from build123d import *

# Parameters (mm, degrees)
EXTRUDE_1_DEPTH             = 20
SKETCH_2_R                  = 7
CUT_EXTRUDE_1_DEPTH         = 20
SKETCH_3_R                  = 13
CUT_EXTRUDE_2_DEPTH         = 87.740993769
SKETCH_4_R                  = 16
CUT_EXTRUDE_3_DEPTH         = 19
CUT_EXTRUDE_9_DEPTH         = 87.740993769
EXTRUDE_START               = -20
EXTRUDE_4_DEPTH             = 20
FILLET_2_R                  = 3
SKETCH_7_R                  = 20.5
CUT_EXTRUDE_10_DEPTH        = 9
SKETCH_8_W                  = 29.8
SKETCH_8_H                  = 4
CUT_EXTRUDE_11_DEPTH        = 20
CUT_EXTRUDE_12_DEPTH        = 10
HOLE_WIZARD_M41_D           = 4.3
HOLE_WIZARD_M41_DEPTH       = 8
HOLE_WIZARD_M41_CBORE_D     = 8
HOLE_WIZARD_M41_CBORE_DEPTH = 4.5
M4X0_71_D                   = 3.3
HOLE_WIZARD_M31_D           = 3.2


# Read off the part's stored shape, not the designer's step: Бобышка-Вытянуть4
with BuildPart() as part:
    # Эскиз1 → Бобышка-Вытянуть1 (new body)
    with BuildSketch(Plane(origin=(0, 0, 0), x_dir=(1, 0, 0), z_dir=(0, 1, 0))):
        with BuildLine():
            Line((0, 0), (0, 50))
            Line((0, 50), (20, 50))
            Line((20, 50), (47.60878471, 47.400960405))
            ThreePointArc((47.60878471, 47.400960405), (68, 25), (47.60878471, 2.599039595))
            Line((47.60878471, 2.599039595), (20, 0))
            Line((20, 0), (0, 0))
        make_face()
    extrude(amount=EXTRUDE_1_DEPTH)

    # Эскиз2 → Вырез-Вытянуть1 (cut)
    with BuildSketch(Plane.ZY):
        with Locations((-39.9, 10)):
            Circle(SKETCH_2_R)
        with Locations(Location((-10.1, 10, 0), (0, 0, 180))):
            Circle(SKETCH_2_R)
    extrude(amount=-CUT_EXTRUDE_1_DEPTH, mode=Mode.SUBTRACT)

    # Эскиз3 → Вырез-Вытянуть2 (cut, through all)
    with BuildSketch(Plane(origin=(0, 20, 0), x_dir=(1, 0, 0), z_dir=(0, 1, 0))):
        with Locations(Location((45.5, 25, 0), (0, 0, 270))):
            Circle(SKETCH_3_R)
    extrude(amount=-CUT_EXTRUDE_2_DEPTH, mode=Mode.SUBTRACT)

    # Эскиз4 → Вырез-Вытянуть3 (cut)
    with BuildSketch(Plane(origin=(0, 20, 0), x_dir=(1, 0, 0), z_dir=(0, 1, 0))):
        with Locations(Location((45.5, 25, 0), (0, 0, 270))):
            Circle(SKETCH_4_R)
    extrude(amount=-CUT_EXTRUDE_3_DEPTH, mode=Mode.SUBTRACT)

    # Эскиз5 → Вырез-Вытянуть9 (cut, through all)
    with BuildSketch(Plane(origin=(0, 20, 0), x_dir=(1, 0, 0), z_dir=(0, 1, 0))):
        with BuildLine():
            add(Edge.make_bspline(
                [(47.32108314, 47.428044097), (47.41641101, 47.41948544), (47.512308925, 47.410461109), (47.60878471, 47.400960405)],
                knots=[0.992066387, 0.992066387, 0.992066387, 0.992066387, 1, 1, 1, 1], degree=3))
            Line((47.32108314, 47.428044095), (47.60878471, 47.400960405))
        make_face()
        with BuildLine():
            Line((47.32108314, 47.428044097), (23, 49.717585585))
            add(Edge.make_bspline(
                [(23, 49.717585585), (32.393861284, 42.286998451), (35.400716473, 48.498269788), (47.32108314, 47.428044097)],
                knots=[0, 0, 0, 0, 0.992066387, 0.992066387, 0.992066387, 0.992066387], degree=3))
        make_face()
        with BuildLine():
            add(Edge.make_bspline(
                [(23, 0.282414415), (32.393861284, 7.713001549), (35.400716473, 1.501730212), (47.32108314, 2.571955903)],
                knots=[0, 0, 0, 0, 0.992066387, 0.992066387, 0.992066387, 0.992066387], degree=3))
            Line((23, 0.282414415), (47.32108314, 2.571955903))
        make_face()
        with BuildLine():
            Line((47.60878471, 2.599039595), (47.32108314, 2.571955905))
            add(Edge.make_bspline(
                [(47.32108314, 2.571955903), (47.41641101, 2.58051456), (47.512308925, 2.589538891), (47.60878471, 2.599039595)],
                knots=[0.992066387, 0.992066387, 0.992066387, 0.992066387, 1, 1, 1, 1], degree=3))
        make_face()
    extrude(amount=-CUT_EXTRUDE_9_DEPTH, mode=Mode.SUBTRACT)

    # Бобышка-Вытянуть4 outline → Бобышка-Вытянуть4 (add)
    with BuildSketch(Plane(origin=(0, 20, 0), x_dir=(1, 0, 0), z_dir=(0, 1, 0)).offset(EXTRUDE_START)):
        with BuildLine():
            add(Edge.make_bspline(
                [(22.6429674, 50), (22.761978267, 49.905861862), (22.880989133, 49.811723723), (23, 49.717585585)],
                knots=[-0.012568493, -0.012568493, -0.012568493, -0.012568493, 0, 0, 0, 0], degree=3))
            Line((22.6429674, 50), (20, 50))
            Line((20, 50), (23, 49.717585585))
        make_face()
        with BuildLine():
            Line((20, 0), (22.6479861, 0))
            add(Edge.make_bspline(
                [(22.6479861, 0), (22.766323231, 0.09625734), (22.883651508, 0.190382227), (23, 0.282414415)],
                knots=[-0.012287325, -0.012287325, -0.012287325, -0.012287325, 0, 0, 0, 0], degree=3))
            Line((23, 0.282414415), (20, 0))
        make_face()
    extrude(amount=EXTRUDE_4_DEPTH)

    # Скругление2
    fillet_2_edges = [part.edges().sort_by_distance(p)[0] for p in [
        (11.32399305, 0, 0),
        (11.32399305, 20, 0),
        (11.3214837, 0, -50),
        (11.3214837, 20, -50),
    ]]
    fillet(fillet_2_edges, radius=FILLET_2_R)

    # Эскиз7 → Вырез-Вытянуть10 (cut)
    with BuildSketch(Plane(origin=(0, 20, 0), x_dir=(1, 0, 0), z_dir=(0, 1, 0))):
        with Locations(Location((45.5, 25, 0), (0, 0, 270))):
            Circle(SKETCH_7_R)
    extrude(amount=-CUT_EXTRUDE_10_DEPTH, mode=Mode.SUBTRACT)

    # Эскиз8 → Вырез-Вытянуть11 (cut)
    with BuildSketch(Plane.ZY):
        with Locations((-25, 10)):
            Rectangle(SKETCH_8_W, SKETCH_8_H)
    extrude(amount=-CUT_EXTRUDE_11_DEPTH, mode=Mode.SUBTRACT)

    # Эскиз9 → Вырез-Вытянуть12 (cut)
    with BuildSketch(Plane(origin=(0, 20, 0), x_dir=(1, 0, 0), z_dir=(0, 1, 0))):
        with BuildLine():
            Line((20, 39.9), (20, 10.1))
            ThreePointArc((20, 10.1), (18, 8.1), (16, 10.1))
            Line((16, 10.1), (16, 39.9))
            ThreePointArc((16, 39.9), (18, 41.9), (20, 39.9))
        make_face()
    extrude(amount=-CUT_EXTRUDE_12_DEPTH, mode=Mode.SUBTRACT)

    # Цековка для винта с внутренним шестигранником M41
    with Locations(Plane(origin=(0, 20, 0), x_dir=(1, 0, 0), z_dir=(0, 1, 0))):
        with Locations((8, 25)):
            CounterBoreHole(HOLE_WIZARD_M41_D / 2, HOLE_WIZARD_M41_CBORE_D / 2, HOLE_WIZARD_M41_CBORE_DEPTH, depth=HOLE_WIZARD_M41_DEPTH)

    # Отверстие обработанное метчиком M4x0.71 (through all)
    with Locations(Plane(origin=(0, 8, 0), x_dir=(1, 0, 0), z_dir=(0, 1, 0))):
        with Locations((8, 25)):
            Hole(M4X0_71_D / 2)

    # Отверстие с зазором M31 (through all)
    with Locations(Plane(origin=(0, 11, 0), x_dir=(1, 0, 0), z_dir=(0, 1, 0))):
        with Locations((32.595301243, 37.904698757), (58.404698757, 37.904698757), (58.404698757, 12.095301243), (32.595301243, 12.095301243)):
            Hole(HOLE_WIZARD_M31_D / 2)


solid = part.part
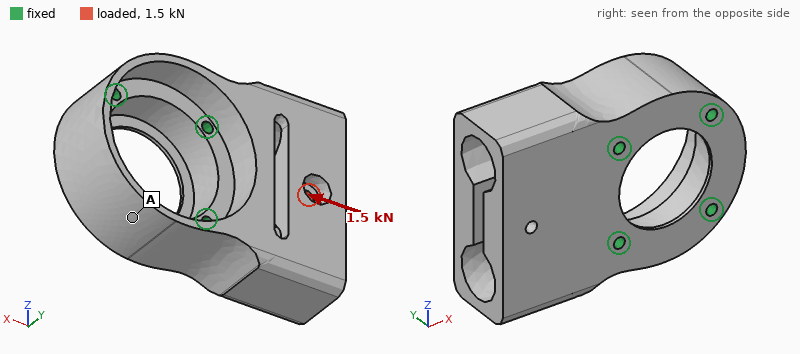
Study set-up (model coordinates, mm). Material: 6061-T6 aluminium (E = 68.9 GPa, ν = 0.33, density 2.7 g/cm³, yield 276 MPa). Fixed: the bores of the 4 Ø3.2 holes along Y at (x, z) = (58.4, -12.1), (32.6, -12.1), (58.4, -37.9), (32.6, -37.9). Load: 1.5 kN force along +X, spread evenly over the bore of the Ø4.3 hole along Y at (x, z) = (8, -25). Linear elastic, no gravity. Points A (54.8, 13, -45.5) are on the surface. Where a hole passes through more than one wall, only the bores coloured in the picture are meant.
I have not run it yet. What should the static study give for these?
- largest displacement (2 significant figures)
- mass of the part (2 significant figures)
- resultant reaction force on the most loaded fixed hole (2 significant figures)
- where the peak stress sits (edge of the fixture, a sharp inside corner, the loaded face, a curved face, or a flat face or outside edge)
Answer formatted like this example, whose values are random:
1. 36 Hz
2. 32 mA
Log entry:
1. 68 µm
2. 79 g
3. 620 N
4. a curved face
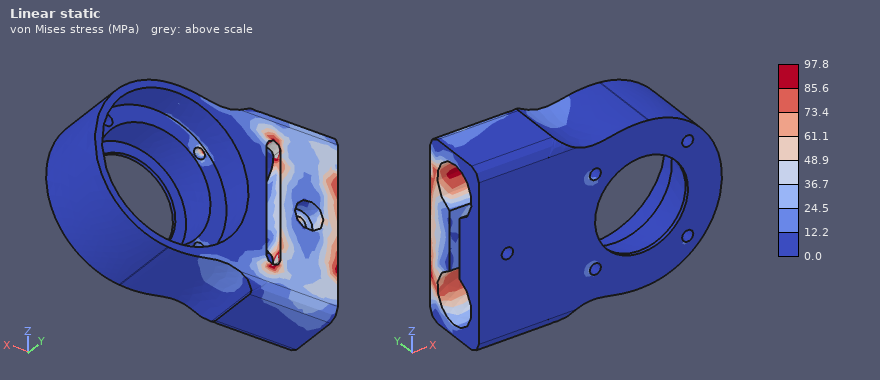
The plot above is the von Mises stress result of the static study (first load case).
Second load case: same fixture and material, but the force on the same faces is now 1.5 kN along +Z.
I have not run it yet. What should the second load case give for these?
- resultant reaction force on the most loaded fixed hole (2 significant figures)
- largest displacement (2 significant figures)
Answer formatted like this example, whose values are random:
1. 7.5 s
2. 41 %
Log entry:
1. 1.2 kN
2. 40 µm
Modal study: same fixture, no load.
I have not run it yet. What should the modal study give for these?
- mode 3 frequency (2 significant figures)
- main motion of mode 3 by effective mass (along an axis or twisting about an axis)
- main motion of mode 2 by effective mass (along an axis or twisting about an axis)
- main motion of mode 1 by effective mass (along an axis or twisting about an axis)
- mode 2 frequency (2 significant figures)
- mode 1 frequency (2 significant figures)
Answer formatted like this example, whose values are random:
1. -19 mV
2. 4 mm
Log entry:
1. 9800 Hz
2. along Z
3. twisting about X
4. along Y
5. 9300 Hz
6. 6000 Hz
